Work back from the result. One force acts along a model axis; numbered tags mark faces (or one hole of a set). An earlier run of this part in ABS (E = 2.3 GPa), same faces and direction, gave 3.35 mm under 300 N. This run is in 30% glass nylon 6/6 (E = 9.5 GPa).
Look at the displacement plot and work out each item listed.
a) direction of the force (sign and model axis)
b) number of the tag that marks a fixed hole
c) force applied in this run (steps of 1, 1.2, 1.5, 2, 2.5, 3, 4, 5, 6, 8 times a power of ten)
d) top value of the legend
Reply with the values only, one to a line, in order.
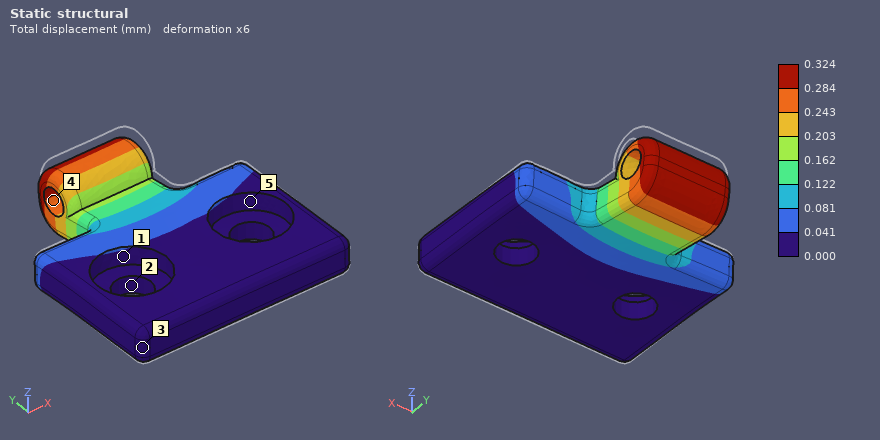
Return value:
-Z
2
120 N
0.324 mm
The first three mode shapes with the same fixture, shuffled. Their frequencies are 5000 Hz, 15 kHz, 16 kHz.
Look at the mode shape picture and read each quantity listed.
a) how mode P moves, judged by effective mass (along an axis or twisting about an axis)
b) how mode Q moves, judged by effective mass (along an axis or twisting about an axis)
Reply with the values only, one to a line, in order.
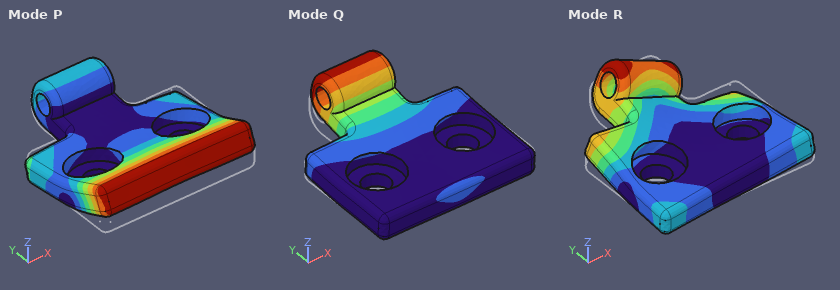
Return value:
along Z
along Z
